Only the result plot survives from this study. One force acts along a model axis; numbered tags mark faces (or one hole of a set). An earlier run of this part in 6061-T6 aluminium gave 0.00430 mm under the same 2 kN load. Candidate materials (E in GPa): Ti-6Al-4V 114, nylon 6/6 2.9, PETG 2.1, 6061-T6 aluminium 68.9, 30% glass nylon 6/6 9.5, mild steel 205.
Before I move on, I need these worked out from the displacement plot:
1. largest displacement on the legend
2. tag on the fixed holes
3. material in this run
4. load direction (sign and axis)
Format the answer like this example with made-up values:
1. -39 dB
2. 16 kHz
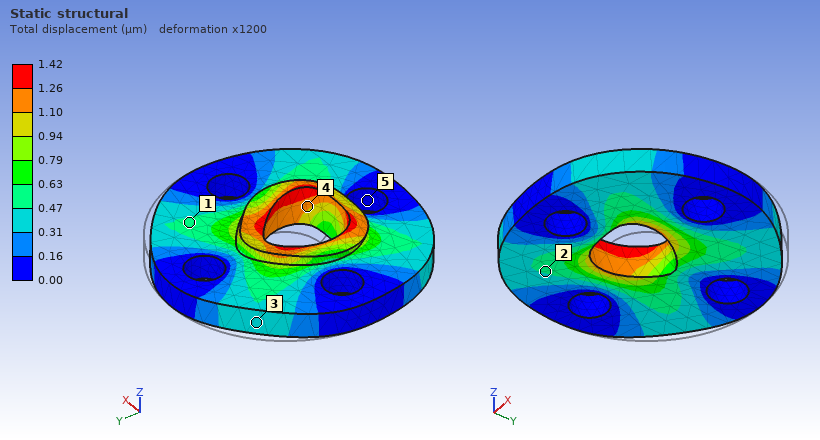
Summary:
1. 1.42 µm
2. 5
3. mild steel
4. -Y
